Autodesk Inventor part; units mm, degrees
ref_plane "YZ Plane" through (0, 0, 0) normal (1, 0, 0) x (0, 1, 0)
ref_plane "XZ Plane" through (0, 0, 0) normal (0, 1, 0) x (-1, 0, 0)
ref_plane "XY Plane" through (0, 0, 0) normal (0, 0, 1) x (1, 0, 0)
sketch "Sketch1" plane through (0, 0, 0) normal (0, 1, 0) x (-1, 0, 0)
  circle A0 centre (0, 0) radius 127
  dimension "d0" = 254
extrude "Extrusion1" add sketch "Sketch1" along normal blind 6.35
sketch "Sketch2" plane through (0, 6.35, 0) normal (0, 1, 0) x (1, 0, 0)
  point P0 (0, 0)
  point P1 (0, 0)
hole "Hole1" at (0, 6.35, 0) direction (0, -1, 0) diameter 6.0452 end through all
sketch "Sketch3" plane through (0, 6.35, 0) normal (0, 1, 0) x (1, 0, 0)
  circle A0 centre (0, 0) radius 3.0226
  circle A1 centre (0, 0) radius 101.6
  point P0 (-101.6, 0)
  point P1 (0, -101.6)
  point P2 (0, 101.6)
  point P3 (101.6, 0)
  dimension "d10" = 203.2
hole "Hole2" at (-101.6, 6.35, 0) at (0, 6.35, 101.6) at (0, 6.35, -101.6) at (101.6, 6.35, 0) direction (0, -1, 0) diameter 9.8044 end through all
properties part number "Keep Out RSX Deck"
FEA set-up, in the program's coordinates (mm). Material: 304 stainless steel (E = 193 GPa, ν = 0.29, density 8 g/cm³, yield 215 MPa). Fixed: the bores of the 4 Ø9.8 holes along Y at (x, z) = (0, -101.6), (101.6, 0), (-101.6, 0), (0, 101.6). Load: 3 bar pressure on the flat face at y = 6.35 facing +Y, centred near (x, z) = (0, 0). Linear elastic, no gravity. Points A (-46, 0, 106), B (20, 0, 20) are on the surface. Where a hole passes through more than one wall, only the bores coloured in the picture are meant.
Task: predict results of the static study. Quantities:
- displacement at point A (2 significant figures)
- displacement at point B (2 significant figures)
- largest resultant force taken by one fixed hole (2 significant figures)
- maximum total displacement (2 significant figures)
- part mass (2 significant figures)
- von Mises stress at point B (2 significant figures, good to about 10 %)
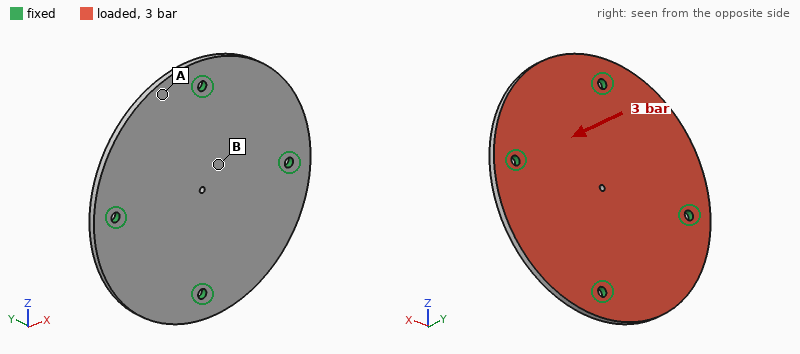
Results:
0.072 mm
0.16 mm
3.8 kN
0.17 mm
2.6 kg
34 MPa
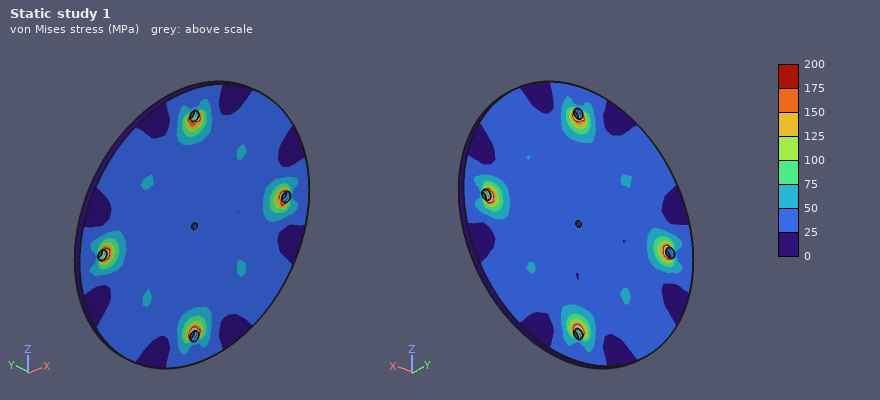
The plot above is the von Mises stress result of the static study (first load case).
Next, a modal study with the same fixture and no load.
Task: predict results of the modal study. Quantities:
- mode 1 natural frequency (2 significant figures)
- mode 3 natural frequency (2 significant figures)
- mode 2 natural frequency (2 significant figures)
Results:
1100 Hz
1200 Hz
1100 Hz
